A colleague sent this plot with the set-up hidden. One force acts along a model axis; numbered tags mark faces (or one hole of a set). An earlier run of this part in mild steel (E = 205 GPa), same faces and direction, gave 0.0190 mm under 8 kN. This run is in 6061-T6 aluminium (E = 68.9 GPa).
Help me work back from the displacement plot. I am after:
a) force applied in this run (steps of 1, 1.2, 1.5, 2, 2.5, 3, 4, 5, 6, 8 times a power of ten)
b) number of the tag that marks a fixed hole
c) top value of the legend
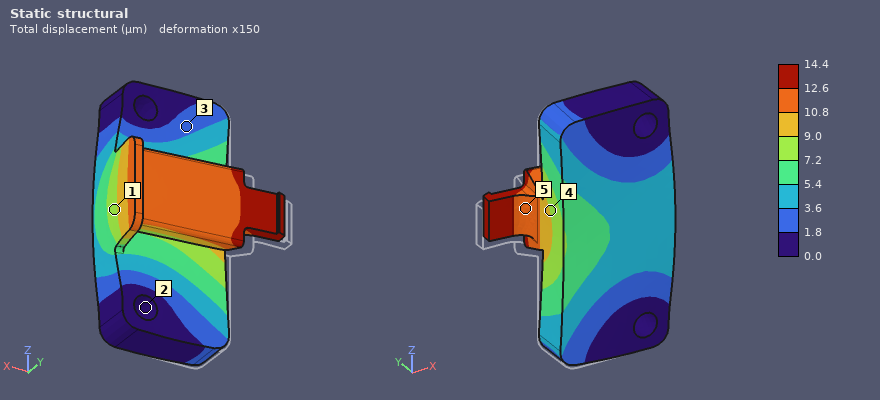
2 kN
2
14.4 µm
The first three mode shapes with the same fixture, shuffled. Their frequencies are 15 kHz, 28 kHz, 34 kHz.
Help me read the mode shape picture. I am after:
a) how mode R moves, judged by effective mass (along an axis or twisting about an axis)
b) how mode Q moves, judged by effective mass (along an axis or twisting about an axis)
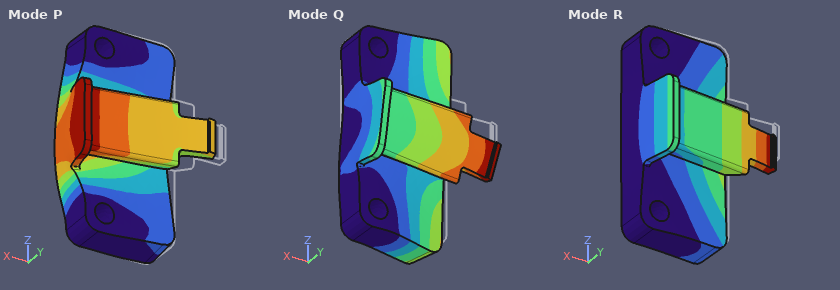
along Y
along Z
